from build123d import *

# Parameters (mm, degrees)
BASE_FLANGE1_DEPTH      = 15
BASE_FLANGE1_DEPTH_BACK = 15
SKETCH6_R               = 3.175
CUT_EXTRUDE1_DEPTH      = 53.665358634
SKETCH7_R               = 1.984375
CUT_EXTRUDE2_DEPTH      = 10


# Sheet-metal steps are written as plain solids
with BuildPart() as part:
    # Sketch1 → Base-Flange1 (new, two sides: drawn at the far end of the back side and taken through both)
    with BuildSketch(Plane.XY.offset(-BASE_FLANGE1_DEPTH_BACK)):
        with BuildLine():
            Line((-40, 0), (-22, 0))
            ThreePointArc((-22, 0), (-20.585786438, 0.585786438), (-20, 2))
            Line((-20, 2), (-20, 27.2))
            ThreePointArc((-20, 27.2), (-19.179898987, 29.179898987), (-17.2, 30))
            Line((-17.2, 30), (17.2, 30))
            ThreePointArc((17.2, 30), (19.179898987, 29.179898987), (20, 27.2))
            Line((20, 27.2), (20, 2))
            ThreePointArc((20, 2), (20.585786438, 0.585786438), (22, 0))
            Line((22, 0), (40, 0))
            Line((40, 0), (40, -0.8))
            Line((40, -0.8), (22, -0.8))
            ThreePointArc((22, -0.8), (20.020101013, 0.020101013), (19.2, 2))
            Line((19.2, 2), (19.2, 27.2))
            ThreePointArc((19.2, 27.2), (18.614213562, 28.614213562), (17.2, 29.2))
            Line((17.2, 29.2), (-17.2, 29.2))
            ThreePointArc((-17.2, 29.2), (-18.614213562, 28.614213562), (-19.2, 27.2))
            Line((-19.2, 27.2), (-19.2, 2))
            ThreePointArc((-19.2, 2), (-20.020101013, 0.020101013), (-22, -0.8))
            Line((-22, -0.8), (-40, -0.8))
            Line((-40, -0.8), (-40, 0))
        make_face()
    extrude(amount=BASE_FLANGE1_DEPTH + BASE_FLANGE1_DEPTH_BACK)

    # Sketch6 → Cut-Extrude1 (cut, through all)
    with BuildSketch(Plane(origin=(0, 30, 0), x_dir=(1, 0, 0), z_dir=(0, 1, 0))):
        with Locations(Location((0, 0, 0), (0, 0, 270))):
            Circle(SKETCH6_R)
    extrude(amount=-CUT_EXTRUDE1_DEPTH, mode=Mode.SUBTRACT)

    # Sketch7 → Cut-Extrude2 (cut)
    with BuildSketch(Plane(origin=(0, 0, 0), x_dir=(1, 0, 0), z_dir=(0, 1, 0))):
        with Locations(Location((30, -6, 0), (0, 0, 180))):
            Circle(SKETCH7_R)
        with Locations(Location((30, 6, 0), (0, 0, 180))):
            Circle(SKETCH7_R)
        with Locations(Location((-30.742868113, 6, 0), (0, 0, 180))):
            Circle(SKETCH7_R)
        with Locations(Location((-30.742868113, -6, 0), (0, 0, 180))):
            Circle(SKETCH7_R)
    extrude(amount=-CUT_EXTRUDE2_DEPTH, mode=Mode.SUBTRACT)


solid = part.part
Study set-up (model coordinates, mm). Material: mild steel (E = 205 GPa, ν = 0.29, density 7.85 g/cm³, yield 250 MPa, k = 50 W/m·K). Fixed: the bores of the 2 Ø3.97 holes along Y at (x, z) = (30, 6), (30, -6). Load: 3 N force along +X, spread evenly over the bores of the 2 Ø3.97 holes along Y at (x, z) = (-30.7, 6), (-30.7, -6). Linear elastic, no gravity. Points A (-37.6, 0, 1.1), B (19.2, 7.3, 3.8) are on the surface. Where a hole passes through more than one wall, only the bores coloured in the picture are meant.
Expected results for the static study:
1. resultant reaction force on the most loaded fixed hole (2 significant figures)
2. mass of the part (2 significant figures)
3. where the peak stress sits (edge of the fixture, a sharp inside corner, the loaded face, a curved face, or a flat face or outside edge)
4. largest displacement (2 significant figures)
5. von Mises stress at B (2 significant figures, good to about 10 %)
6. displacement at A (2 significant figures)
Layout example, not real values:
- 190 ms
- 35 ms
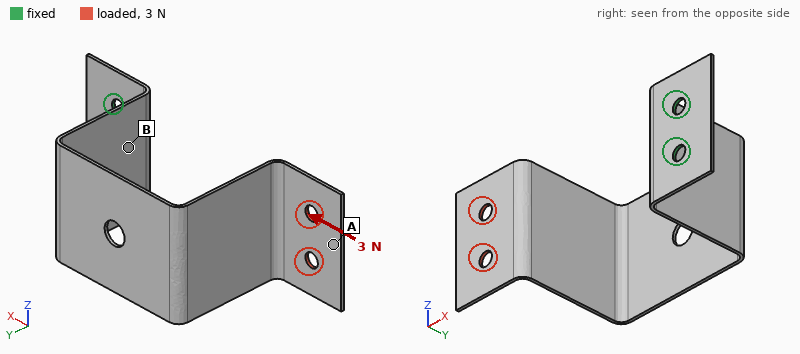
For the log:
- 1.5 N
- 25 g
- a curved face
- 1.1 mm
- 6.6 MPa
- 1.0 mm
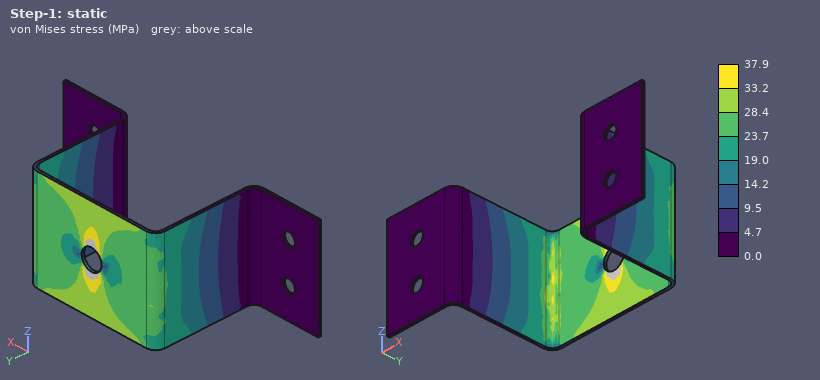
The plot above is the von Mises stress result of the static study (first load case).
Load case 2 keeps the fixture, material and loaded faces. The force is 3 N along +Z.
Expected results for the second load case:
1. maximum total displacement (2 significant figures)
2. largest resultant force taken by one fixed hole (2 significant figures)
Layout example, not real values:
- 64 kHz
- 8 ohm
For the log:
- 0.87 mm
- 12 N
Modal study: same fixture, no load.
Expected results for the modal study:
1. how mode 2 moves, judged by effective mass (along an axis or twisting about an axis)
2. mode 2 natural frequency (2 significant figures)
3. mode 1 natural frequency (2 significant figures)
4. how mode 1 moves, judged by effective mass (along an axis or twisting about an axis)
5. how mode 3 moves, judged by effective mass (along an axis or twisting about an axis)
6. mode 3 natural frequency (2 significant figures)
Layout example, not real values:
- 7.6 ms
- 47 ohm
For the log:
- along Z
- 120 Hz
- 73 Hz
- along Y
- along X
- 170 Hz
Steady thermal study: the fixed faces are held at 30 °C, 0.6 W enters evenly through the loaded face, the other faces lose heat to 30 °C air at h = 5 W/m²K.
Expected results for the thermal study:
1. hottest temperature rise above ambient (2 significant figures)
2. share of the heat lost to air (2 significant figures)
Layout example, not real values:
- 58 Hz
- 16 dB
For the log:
- 28 K
- 74 %
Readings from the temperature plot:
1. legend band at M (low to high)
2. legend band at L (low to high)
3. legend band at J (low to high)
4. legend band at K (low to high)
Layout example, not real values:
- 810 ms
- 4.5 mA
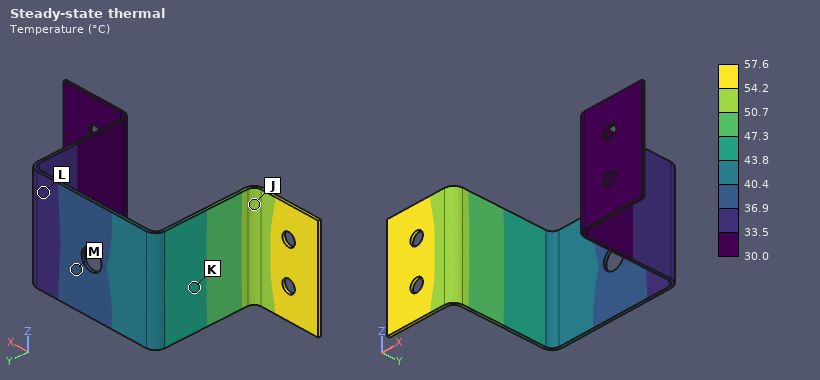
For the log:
- 36.9 to 40.4 °C
- 33.5 to 36.9 °C
- 50.7 to 54.2 °C
- 43.8 to 47.3 °C
